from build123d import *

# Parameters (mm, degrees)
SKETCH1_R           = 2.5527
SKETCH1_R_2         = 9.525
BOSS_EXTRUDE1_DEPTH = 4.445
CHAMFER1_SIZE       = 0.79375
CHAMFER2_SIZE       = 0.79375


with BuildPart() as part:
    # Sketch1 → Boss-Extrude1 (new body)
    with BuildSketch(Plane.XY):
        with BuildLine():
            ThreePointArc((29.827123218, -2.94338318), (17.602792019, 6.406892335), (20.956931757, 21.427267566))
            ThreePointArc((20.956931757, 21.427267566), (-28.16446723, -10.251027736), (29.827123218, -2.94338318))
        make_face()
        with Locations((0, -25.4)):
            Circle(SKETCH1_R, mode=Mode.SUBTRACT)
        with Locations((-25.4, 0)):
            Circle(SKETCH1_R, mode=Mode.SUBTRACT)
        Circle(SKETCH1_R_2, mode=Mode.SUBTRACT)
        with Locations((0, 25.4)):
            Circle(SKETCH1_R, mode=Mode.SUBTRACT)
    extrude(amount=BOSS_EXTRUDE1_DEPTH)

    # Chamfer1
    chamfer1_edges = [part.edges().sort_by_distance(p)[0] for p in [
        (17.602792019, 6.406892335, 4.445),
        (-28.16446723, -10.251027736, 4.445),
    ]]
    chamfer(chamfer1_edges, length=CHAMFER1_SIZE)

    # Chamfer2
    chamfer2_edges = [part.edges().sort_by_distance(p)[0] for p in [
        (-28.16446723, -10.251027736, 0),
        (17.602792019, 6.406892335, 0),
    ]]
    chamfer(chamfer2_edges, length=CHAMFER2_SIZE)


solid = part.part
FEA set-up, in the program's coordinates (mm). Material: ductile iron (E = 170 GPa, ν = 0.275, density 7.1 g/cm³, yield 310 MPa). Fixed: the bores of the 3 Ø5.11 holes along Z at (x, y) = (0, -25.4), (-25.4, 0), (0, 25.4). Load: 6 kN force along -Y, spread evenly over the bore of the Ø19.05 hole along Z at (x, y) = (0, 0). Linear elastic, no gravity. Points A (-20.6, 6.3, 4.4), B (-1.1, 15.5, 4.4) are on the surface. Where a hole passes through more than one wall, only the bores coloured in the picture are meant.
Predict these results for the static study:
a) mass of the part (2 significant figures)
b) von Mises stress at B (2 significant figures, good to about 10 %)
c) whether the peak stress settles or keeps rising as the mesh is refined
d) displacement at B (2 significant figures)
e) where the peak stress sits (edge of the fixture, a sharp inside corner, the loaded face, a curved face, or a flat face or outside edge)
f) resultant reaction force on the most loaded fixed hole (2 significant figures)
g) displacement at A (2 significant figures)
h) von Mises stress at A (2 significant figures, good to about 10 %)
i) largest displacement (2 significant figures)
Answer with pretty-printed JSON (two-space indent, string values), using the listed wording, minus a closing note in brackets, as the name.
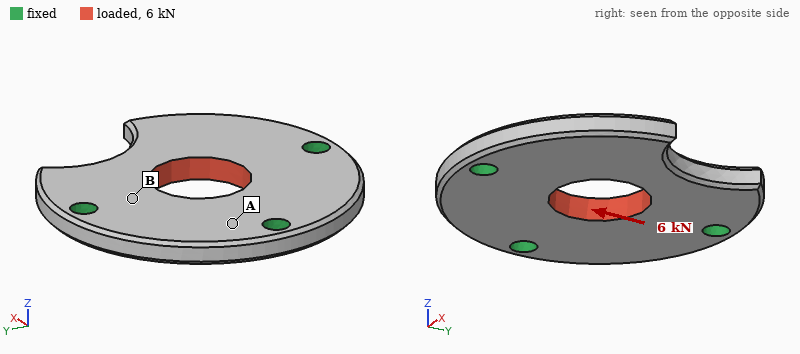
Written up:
{
  "mass of the part": "71 g",
  "von Mises stress at B": "35 MPa",
  "whether the peak stress settles or keeps rising as the mesh is refined": "keeps rising",
  "displacement at B": "1.9 µm",
  "where the peak stress sits": "edge of the fixture",
  "resultant reaction force on the most loaded fixed hole": "2.5 kN",
  "displacement at A": "1.1 µm",
  "von Mises stress at A": "14 MPa",
  "largest displacement": "5.4 µm"
}
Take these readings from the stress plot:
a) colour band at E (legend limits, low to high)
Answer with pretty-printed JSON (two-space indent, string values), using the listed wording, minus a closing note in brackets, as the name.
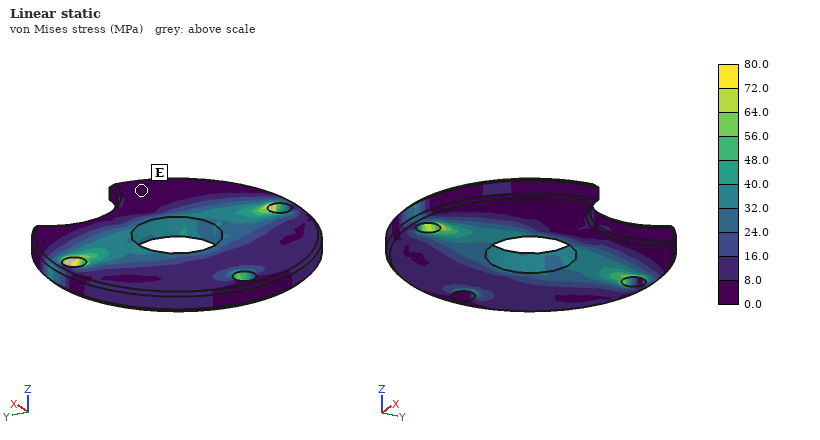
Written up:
{
  "colour band at E": "0.0 to 8.0 MPa"
}
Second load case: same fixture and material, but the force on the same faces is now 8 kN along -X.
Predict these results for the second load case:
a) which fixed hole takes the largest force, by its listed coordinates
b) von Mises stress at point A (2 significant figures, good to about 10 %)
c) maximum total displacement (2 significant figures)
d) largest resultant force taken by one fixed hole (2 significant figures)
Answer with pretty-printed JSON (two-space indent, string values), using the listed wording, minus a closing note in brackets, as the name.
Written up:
{
  "which fixed hole takes the largest force, by its listed coordinates": "(-25.4, 0)",
  "von Mises stress at point A": "35 MPa",
  "maximum total displacement": "12 µm",
  "largest resultant force taken by one fixed hole": "3.1 kN"
}
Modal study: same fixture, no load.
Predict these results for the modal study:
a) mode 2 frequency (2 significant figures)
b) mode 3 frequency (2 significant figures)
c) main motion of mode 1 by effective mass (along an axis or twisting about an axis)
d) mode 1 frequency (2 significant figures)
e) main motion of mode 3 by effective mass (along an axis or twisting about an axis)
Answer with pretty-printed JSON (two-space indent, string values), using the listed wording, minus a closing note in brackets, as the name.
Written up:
{
  "mode 2 frequency": "11 kHz",
  "mode 3 frequency": "15 kHz",
  "main motion of mode 1 by effective mass": "along Z",
  "mode 1 frequency": "4500 Hz",
  "main motion of mode 3 by effective mass": "along Z"
}
